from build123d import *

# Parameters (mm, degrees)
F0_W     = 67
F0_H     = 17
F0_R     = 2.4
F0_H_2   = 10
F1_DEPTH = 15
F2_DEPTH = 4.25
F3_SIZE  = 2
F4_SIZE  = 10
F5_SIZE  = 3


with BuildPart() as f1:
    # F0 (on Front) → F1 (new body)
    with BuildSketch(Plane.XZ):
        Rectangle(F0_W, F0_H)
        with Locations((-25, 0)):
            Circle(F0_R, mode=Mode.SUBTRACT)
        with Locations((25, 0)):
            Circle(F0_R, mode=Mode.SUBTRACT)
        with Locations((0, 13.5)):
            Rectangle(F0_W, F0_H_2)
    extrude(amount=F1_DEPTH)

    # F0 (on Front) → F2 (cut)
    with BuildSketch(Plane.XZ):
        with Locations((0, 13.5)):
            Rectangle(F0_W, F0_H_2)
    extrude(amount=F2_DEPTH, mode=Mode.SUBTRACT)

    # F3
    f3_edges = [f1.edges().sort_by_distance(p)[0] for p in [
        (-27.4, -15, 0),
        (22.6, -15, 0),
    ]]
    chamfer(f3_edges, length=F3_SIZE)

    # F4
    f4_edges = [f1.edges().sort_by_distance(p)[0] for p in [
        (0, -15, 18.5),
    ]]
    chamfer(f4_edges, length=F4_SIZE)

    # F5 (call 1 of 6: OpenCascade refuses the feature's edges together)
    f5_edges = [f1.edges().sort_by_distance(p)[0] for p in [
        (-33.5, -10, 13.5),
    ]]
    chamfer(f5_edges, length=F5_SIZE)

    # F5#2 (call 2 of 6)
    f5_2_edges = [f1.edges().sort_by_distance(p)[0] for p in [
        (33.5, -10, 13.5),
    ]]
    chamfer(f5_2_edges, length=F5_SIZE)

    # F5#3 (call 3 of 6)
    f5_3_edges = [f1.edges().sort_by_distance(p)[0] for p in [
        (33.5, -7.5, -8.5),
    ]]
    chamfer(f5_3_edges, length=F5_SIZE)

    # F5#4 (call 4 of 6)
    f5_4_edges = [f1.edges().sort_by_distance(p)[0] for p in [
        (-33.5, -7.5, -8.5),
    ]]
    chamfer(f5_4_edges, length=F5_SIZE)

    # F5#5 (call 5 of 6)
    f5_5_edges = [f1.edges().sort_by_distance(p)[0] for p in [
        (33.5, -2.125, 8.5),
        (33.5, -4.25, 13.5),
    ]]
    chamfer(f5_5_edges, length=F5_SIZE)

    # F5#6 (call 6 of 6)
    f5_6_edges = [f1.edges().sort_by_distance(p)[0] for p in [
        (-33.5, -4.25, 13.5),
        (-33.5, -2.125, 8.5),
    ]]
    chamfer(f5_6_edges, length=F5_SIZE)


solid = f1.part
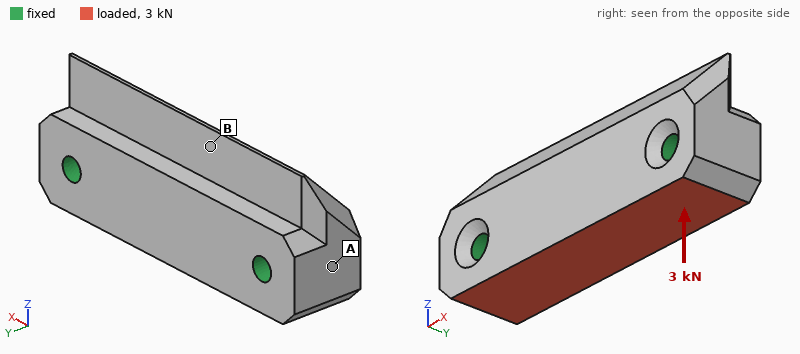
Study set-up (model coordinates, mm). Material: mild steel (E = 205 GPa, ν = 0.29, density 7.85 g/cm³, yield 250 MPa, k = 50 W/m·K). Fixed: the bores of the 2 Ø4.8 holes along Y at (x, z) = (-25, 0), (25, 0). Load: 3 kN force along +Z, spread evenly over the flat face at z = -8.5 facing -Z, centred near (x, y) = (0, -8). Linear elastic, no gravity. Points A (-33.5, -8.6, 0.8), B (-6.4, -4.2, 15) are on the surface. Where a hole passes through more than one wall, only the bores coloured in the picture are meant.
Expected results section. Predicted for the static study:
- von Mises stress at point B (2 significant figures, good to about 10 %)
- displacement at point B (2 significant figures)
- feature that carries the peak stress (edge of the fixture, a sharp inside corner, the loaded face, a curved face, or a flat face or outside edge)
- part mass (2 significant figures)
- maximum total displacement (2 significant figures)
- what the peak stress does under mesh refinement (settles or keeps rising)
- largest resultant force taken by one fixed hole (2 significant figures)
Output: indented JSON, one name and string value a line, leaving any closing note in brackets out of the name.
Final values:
{
  "von Mises stress at point B": "8.3 MPa",
  "displacement at point B": "1.3 µm",
  "feature that carries the peak stress": "edge of the fixture",
  "part mass": "160 g",
  "maximum total displacement": "1.6 µm",
  "what the peak stress does under mesh refinement": "keeps rising",
  "largest resultant force taken by one fixed hole": "1.5 kN"
}
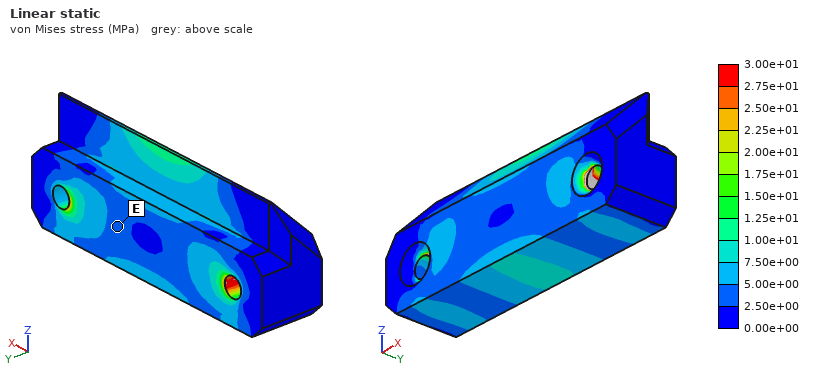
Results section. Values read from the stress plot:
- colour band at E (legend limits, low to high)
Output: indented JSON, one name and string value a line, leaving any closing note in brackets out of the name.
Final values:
{
  "colour band at E": "2.50e+00 to 5.00e+00 MPa"
}
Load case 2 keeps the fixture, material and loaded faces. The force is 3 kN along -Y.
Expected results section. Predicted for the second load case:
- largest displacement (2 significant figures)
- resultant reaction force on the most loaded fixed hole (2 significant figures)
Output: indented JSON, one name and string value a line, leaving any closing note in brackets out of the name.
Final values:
{
  "largest displacement": "4.2 µm",
  "resultant reaction force on the most loaded fixed hole": "1.5 kN"
}
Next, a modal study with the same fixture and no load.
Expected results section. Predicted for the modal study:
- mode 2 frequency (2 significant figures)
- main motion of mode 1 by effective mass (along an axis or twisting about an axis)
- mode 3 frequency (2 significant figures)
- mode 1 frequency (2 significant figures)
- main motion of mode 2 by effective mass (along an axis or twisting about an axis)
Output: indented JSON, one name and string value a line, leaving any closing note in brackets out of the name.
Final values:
{
  "mode 2 frequency": "20 kHz",
  "main motion of mode 1 by effective mass": "along Y",
  "mode 3 frequency": "24 kHz",
  "mode 1 frequency": "18 kHz",
  "main motion of mode 2 by effective mass": "along Z"
}
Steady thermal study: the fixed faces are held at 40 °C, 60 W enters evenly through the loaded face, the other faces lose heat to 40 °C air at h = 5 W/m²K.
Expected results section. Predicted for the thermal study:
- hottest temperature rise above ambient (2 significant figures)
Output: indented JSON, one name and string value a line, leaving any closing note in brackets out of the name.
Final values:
{
  "hottest temperature rise above ambient": "31 K"
}
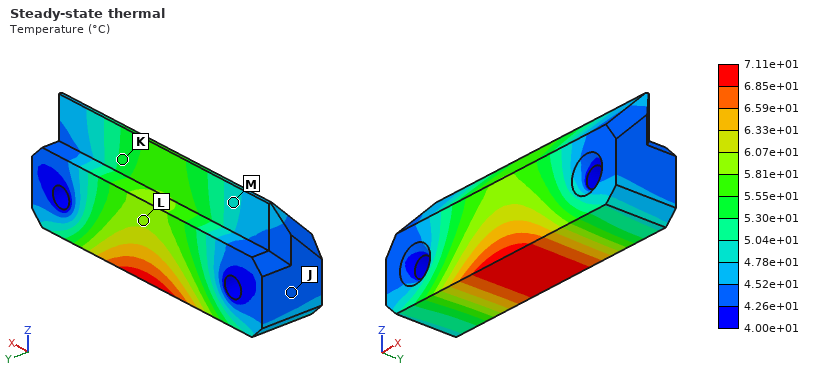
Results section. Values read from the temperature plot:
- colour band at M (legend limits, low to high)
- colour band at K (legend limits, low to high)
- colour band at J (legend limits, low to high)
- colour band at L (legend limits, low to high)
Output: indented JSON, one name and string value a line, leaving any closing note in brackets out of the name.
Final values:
{
  "colour band at M": "4.78e+01 to 5.04e+01 °C",
  "colour band at K": "5.30e+01 to 5.55e+01 °C",
  "colour band at J": "4.26e+01 to 4.52e+01 °C",
  "colour band at L": "5.81e+01 to 6.07e+01 °C"
}
